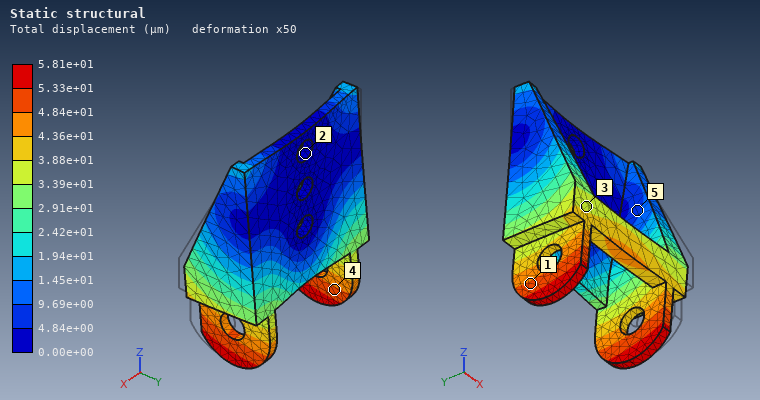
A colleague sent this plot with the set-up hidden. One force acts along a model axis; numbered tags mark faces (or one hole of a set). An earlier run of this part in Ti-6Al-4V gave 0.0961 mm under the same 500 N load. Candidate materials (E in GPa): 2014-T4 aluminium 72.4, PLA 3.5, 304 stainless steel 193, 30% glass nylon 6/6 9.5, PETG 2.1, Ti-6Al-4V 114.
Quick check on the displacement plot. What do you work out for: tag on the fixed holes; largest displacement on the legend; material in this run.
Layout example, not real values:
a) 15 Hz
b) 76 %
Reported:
a) 2
b) 5.81e+01 µm
c) 304 stainless steel
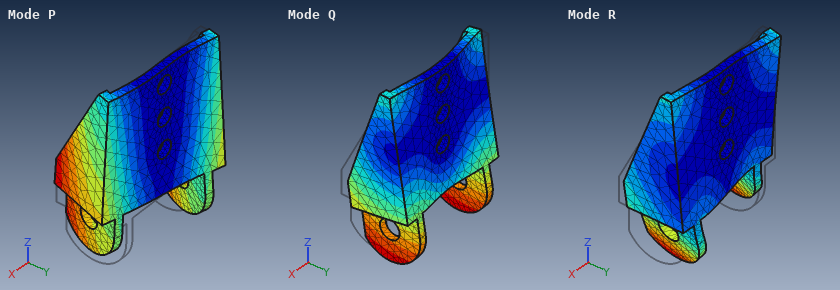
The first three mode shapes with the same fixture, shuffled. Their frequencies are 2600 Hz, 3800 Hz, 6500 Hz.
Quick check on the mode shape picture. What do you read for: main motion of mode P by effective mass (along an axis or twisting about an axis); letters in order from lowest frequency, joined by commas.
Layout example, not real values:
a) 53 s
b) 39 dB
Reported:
a) along X
b) P, Q, R
